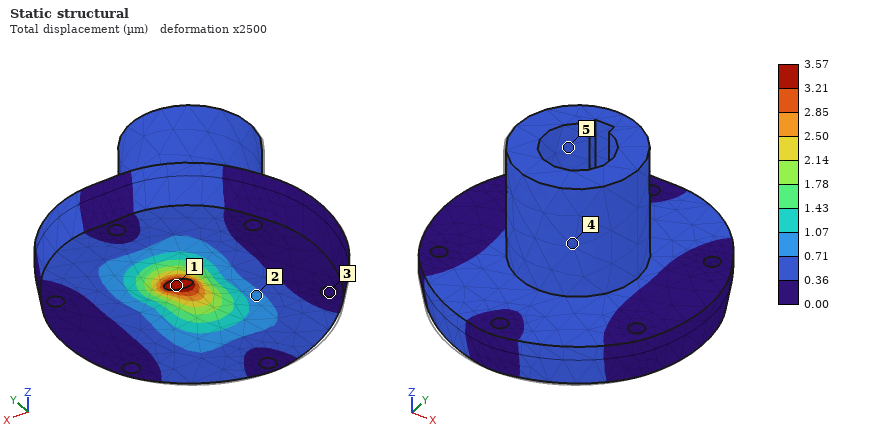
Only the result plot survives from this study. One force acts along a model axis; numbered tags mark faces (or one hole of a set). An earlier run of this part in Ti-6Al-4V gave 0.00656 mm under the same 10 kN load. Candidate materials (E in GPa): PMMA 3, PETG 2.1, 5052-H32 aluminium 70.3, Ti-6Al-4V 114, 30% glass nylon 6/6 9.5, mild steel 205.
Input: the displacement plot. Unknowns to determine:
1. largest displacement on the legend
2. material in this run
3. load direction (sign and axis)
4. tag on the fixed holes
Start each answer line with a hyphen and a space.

- 3.57 µm
- mild steel
- +Y
- 3
